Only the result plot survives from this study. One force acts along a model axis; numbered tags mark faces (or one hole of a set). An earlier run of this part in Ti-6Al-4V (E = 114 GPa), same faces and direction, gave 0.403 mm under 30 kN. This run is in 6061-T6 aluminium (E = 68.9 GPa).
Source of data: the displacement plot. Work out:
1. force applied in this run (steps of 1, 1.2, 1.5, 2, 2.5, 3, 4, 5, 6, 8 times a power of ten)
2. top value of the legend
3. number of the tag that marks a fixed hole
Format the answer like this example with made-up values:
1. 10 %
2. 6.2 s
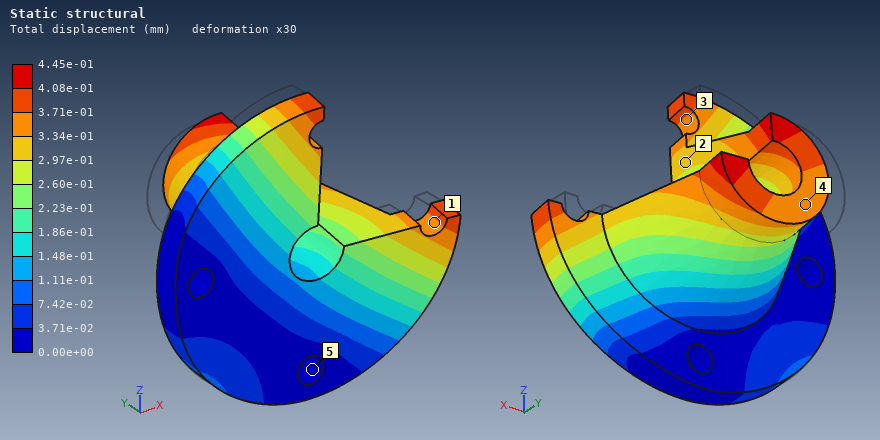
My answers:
1. 20 kN
2. 4.45e-01 mm
3. 5
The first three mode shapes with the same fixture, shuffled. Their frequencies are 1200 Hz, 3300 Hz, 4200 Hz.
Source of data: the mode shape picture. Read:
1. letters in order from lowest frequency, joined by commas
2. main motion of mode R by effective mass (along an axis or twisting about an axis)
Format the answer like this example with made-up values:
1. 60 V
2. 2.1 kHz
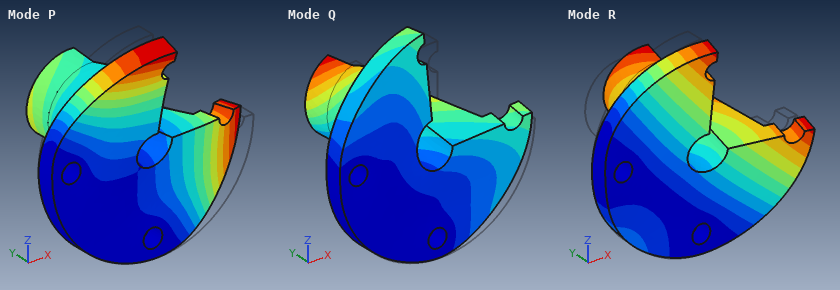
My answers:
1. R, P, Q
2. along Y
